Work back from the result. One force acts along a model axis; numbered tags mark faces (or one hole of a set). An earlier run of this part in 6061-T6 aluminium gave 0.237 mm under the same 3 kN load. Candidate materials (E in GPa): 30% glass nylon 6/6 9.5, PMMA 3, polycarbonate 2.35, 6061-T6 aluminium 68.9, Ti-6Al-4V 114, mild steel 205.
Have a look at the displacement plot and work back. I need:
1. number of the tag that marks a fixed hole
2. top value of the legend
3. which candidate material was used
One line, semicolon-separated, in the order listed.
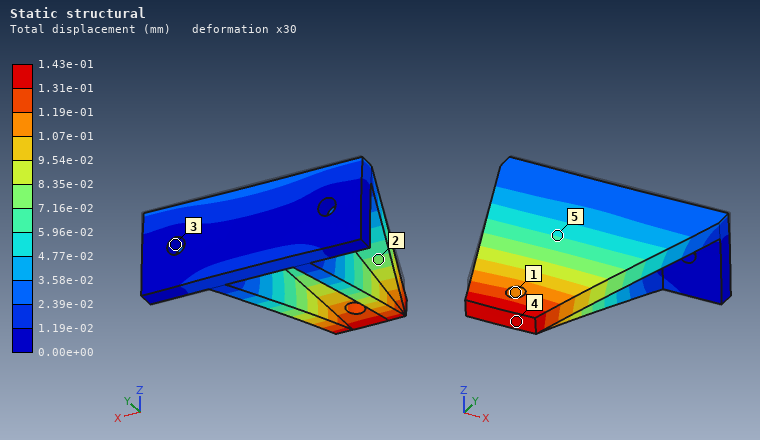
3; 1.43e-01 mm; Ti-6Al-4V
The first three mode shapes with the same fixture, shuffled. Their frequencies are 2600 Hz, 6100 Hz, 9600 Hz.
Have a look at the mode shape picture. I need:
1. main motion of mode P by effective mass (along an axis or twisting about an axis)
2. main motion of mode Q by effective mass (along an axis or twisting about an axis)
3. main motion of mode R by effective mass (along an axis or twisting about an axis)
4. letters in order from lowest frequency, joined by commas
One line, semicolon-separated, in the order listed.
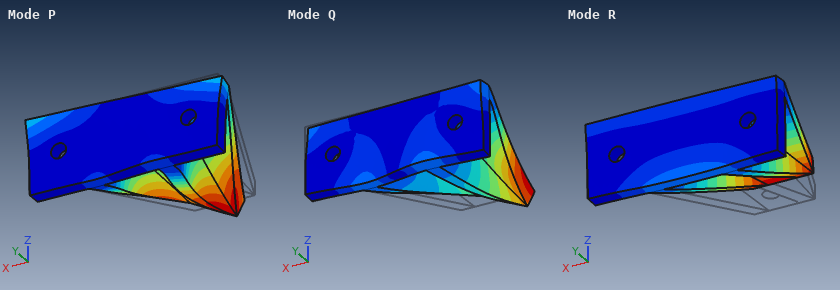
along X; along X; along Z; R, P, Q
